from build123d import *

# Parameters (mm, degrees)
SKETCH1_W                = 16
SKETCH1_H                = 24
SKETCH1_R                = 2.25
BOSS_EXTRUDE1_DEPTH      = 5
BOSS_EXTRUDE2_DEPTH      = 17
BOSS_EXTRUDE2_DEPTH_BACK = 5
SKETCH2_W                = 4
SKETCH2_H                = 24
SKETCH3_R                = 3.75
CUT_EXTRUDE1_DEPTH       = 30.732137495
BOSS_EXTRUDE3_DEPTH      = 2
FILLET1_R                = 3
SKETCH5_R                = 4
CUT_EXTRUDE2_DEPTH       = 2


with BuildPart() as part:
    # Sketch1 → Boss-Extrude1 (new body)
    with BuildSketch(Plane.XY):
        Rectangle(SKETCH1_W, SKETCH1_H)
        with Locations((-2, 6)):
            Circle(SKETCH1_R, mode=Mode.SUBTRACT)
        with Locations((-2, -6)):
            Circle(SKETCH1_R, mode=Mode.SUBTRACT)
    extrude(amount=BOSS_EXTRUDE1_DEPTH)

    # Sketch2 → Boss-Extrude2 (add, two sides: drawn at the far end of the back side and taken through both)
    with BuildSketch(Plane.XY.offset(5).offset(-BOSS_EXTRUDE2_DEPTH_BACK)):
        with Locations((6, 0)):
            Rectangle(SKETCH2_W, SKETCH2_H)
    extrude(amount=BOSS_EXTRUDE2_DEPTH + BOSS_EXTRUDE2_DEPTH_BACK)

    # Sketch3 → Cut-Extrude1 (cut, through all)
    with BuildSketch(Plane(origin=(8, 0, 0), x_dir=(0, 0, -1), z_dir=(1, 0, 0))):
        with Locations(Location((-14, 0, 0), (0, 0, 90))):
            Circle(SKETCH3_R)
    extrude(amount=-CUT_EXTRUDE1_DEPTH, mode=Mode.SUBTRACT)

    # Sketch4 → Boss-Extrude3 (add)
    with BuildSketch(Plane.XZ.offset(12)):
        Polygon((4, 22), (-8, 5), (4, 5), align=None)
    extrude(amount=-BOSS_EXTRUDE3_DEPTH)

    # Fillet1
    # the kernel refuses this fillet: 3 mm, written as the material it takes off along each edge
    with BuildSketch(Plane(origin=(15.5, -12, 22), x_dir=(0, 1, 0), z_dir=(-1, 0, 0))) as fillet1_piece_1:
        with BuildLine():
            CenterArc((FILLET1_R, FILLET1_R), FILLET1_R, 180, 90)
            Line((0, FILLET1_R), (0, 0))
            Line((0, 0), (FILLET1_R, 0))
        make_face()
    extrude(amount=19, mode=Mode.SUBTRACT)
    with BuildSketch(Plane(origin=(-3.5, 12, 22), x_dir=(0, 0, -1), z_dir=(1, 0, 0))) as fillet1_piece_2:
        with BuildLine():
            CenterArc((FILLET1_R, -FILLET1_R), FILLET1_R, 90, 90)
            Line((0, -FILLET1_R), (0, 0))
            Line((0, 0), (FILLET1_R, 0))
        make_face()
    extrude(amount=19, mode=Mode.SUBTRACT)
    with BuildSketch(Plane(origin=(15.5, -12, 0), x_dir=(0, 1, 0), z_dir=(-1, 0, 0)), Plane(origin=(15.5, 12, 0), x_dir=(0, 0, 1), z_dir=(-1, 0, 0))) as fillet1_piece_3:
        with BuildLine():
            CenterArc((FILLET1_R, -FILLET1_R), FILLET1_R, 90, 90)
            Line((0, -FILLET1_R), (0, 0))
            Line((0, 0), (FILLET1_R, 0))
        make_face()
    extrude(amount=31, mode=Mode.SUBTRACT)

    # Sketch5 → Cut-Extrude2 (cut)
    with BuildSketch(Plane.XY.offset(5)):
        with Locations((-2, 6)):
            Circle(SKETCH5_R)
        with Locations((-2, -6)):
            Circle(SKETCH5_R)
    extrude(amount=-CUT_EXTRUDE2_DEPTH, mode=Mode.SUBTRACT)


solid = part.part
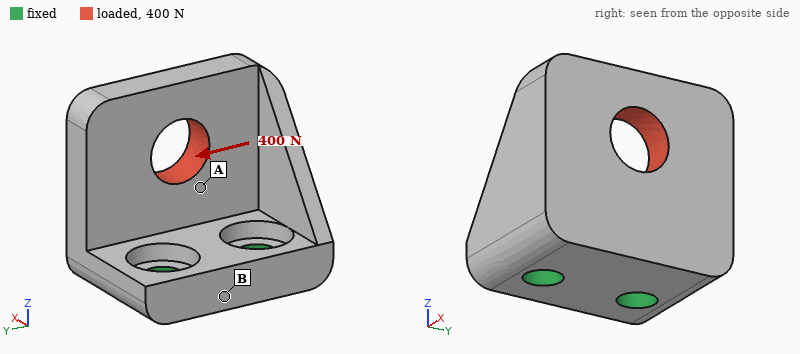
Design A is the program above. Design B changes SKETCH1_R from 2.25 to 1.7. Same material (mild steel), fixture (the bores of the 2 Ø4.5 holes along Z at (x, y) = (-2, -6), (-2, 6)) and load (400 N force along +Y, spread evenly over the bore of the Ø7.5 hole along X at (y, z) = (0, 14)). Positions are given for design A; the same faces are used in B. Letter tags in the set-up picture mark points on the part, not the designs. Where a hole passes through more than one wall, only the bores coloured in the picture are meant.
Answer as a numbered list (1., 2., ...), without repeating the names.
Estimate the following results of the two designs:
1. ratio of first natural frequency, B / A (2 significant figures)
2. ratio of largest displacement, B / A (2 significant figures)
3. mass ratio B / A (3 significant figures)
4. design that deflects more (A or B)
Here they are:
1. 0.90
2. 1.2
3. 1.01
4. B
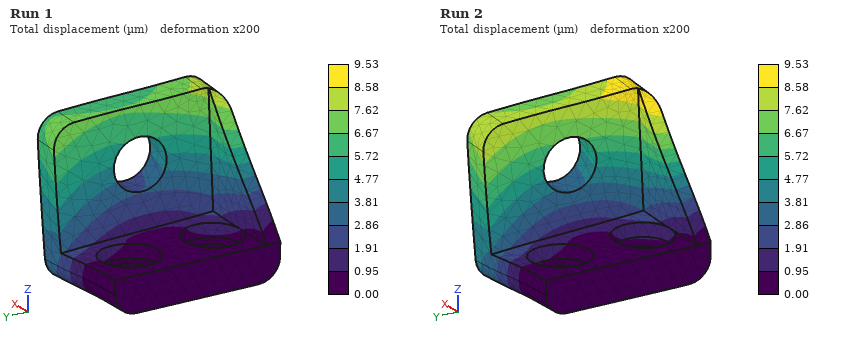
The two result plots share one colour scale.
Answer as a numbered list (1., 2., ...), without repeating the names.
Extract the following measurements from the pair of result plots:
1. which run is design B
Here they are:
1. Run 2
